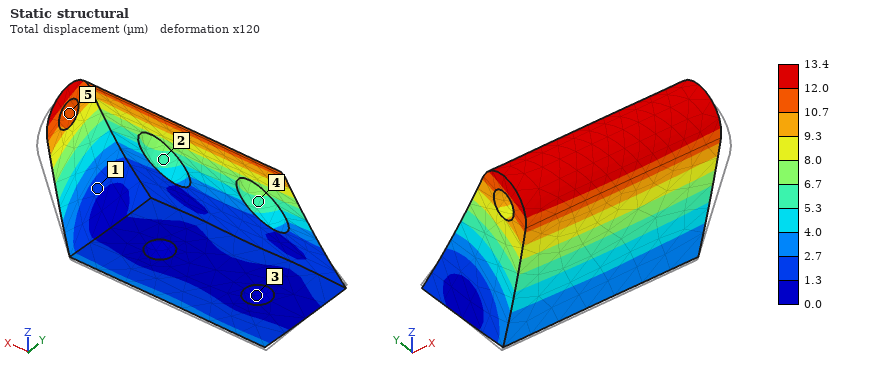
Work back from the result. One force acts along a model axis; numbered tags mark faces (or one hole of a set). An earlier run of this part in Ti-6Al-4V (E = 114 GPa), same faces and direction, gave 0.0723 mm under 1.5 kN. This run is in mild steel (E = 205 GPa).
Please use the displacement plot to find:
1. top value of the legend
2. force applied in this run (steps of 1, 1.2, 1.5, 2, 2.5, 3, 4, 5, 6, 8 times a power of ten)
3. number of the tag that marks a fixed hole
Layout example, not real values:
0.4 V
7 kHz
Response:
13.4 µm
500 N
3
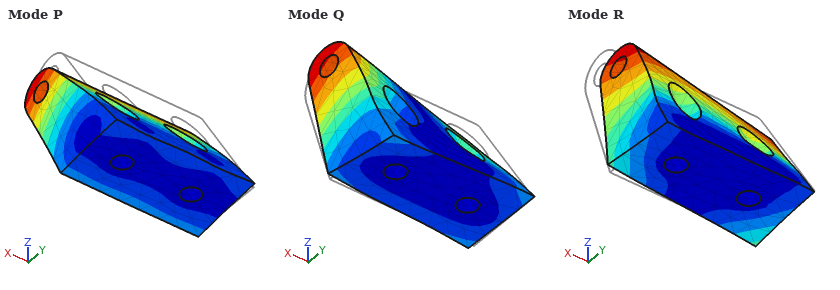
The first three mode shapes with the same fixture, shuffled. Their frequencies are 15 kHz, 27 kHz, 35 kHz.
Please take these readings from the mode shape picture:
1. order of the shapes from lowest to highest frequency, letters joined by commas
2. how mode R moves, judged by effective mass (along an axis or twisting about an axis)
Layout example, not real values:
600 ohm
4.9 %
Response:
P, R, Q
along X
